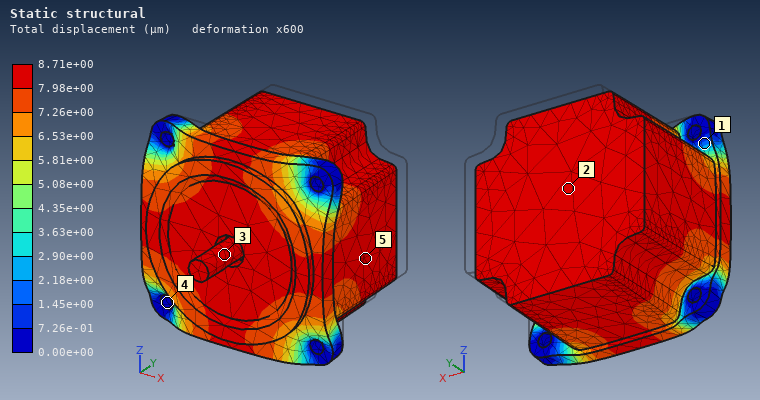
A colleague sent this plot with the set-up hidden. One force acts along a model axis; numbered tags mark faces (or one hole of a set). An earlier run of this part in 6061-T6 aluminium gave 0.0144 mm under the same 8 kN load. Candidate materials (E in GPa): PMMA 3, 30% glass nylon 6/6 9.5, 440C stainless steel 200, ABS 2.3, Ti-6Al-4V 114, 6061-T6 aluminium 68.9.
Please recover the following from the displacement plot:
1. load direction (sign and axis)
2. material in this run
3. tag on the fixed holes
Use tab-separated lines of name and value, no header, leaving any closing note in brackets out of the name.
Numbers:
load direction	-Y
material in this run	Ti-6Al-4V
tag on the fixed holes	4
